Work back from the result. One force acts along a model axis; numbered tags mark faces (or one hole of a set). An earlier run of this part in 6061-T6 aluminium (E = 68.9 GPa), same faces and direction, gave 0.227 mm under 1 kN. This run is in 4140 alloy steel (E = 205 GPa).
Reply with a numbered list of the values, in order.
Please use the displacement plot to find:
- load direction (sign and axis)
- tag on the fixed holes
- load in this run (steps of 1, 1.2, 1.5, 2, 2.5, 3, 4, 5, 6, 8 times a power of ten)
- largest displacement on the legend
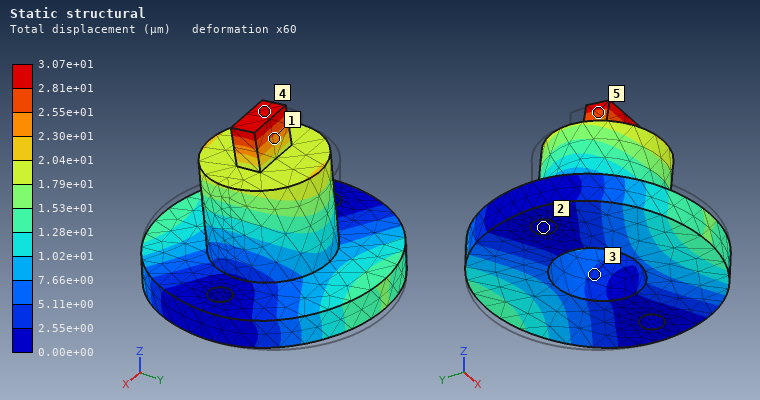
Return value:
1. -Y
2. 2
3. 400 N
4. 3.07e+01 µm
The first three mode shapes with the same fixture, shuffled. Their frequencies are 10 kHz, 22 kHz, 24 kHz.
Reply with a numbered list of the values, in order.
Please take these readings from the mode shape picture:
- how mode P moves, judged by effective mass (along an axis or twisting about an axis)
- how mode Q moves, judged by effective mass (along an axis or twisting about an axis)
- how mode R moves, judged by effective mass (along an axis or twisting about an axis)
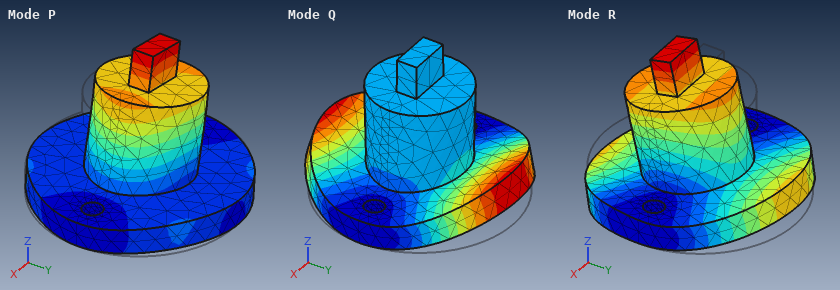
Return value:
1. along X
2. along Z
3. along Y
